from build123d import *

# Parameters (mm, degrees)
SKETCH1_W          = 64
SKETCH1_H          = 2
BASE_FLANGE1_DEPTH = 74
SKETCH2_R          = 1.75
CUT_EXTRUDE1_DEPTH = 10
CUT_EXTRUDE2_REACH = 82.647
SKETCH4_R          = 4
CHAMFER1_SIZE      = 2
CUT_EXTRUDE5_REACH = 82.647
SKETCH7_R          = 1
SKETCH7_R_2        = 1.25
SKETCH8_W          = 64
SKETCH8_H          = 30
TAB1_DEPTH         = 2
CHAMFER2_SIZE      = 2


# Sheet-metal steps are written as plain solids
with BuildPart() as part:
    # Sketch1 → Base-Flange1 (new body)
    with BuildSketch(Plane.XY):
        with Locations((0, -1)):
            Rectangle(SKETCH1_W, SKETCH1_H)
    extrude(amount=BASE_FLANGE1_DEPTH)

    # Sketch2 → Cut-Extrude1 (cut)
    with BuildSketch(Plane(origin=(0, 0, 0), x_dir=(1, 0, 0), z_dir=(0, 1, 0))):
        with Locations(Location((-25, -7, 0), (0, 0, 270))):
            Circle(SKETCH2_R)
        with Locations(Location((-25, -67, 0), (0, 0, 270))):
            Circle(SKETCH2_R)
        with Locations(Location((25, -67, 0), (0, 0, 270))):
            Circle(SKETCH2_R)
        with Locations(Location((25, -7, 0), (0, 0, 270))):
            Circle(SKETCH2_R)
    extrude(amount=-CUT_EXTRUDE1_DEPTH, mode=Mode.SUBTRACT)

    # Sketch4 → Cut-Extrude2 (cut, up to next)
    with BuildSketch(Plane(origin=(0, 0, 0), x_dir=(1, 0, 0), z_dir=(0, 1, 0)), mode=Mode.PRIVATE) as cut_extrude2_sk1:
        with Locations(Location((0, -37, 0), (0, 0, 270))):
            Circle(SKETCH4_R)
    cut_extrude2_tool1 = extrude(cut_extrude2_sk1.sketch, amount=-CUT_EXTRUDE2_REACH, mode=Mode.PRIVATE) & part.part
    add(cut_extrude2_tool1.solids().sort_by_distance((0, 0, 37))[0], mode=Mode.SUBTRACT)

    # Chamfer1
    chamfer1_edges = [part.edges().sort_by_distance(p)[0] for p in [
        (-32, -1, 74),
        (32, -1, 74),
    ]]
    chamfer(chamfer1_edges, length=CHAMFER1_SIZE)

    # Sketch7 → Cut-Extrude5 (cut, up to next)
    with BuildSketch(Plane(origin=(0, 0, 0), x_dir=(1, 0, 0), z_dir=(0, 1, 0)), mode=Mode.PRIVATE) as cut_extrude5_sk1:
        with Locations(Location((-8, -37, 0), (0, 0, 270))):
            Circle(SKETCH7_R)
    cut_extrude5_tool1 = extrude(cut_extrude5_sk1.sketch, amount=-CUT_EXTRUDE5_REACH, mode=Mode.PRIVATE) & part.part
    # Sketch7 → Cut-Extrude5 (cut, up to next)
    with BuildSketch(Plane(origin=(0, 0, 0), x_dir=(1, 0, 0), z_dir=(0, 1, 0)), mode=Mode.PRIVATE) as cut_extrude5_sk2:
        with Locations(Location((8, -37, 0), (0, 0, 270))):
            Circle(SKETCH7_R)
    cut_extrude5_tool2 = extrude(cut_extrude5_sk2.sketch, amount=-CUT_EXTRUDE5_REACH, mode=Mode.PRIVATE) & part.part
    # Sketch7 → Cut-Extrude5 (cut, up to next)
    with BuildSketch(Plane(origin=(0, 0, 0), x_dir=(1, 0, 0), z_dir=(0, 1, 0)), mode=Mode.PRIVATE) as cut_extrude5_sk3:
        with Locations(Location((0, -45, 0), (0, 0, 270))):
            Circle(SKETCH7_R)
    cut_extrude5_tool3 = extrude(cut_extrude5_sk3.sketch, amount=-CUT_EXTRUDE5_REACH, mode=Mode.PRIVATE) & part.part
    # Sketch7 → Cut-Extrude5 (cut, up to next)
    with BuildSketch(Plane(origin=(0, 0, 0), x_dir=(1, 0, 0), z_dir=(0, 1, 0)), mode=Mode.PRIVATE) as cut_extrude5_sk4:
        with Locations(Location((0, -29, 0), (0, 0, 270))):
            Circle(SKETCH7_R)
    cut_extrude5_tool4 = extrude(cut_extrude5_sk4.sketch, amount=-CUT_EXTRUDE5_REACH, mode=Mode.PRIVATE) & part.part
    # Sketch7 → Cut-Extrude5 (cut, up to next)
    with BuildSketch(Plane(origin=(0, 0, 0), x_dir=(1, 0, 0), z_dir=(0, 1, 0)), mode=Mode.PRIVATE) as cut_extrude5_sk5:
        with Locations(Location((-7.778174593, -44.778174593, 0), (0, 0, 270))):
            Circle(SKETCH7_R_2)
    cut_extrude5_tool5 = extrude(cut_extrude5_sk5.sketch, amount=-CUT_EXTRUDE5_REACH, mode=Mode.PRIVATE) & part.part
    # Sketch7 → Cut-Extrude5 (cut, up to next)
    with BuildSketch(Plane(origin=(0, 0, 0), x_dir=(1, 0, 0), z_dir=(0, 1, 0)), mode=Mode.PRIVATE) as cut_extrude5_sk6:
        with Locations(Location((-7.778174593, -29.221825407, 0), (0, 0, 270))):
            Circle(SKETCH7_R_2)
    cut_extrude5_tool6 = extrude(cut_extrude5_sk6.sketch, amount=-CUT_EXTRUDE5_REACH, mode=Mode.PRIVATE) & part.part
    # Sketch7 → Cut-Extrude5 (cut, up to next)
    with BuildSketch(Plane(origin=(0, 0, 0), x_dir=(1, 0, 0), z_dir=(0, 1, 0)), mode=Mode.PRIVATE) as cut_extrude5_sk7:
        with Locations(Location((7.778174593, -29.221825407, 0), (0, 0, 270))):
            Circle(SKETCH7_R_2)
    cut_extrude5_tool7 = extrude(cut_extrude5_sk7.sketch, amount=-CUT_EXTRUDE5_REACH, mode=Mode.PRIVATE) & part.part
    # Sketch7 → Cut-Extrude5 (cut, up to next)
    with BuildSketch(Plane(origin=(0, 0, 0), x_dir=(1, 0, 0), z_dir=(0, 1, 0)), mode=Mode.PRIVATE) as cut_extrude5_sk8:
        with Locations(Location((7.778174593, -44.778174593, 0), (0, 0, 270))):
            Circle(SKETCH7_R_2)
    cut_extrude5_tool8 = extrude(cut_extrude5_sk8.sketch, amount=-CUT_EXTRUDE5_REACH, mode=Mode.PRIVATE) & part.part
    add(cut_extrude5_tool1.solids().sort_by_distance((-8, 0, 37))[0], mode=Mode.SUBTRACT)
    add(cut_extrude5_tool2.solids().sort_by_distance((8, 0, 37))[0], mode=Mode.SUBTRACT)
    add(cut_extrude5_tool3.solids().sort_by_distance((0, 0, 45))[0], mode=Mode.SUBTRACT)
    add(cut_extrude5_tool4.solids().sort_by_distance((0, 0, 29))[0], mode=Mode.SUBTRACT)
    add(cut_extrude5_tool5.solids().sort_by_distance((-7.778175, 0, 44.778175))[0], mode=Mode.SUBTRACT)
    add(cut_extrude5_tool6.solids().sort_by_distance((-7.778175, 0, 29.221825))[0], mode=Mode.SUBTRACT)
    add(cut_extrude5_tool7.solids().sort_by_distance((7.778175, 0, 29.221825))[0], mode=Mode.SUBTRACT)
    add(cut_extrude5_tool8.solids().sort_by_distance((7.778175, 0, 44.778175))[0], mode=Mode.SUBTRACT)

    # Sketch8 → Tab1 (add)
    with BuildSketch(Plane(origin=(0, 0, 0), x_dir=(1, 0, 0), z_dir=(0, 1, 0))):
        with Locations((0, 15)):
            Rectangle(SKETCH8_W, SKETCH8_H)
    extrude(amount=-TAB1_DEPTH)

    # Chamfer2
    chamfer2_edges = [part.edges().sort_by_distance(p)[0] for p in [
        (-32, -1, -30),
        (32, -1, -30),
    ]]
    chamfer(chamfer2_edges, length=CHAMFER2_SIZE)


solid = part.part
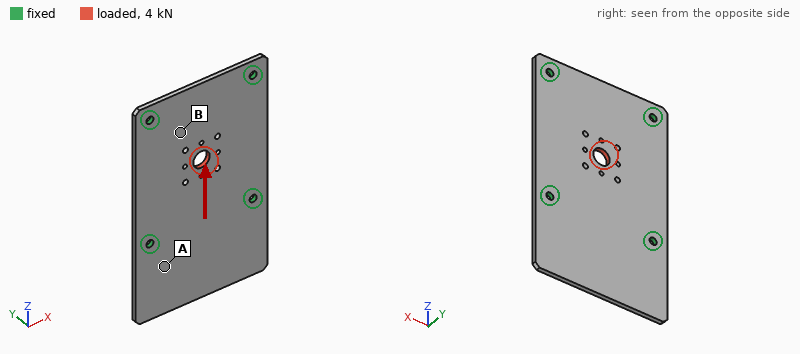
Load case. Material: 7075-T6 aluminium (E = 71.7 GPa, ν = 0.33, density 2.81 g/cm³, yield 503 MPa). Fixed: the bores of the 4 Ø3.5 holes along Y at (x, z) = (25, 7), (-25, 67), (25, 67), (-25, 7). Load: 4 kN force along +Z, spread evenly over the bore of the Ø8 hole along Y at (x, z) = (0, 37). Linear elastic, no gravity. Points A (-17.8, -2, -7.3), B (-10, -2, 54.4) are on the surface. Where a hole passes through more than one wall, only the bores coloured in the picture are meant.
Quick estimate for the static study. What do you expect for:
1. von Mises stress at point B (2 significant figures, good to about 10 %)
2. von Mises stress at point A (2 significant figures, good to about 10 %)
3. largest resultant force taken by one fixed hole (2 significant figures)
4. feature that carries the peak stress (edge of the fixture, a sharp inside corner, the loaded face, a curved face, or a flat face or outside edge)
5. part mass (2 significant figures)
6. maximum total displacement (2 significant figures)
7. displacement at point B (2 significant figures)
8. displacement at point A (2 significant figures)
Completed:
30 MPa
10 MPa
1.1 kN
a curved face
37 g
25 µm
12 µm
4.6 µm
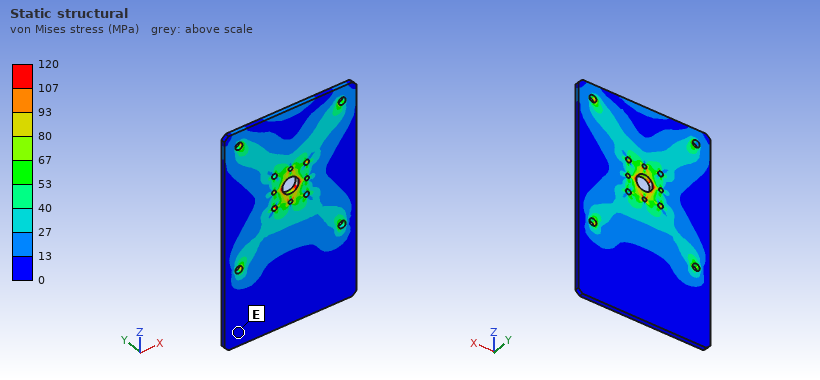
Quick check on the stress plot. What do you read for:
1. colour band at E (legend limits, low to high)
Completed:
0 to 13 MPa
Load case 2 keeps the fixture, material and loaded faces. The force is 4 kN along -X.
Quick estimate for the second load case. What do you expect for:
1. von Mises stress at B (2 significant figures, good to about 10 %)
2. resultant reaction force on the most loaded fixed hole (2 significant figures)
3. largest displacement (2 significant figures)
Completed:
35 MPa
1.2 kN
31 µm
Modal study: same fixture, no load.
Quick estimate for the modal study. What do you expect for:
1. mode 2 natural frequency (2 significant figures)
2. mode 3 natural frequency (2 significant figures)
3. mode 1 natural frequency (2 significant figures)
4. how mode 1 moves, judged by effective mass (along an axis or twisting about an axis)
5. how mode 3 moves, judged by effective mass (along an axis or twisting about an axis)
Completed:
2100 Hz
2300 Hz
1100 Hz
along Y
along Y
